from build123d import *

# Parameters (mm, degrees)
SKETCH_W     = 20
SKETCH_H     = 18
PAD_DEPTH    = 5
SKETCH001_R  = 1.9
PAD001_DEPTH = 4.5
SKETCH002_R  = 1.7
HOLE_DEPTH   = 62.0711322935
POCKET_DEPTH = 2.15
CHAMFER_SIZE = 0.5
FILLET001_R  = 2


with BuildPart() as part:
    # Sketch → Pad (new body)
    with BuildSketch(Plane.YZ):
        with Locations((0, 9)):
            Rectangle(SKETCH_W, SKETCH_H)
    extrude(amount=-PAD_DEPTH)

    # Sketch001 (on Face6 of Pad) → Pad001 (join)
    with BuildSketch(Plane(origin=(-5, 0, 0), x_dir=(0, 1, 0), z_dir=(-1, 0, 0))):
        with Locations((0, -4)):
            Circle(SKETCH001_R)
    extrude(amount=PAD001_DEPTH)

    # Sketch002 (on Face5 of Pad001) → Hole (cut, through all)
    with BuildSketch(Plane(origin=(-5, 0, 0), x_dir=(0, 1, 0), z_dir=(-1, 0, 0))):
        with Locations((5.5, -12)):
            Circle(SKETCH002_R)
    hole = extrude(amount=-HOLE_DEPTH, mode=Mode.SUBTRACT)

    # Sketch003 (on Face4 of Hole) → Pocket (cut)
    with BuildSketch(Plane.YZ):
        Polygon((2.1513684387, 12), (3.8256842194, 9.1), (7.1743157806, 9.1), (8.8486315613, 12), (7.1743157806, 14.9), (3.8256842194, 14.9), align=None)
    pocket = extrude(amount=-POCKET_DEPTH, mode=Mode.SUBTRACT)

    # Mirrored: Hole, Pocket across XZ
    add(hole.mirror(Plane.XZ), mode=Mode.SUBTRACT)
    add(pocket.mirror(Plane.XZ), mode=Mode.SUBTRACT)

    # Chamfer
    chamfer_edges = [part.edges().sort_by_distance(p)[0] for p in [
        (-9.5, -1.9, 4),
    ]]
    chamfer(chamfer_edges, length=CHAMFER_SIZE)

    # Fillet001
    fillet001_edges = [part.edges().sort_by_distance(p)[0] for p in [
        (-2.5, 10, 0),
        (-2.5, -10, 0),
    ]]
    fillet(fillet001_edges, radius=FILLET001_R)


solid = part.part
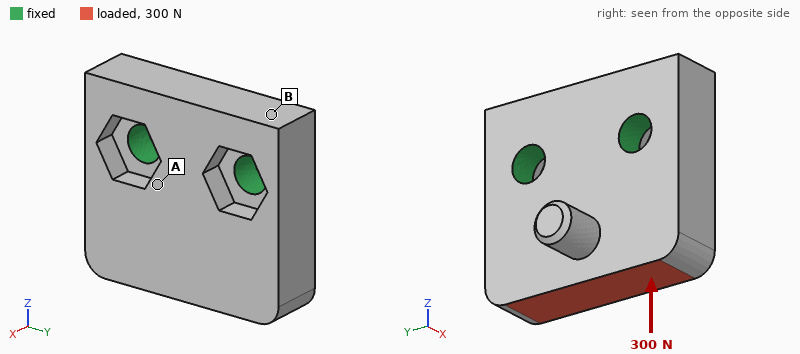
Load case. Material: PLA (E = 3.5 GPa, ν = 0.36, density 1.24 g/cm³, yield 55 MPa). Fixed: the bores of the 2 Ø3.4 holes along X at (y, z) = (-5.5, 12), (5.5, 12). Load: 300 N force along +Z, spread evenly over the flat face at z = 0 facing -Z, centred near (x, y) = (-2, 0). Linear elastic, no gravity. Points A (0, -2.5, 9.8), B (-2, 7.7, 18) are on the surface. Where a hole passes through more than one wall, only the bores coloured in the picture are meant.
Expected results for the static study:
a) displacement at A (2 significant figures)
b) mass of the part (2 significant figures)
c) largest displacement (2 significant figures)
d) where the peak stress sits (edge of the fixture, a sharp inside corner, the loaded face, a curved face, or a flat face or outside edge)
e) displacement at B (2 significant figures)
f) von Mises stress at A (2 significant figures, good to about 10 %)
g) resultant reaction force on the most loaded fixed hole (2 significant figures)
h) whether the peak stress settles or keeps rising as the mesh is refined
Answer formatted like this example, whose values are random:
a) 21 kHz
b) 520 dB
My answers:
a) 16 µm
b) 2.1 g
c) 43 µm
d) edge of the fixture
e) 9.9 µm
f) 3.9 MPa
g) 150 N
h) keeps rising
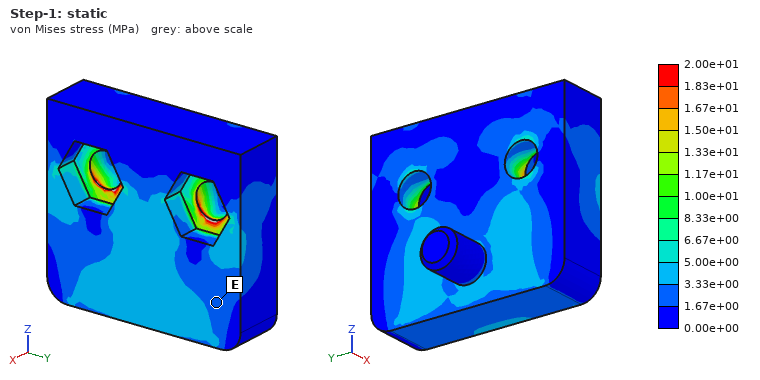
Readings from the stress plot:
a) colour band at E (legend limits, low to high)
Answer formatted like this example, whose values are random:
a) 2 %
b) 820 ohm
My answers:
a) 1.67e+00 to 3.33e+00 MPa
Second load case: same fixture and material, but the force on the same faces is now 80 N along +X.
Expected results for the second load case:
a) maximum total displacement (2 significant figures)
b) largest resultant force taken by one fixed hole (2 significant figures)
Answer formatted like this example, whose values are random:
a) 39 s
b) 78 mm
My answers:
a) 0.14 mm
b) 41 N
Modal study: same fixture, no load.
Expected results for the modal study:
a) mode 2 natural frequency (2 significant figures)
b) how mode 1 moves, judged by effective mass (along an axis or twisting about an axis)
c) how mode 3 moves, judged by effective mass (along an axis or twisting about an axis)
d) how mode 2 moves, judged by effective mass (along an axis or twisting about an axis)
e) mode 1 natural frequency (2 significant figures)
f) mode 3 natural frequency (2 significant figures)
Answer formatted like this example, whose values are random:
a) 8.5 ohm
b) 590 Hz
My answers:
a) 11 kHz
b) along X
c) along Y
d) twisting about Z
e) 5900 Hz
f) 14 kHz
